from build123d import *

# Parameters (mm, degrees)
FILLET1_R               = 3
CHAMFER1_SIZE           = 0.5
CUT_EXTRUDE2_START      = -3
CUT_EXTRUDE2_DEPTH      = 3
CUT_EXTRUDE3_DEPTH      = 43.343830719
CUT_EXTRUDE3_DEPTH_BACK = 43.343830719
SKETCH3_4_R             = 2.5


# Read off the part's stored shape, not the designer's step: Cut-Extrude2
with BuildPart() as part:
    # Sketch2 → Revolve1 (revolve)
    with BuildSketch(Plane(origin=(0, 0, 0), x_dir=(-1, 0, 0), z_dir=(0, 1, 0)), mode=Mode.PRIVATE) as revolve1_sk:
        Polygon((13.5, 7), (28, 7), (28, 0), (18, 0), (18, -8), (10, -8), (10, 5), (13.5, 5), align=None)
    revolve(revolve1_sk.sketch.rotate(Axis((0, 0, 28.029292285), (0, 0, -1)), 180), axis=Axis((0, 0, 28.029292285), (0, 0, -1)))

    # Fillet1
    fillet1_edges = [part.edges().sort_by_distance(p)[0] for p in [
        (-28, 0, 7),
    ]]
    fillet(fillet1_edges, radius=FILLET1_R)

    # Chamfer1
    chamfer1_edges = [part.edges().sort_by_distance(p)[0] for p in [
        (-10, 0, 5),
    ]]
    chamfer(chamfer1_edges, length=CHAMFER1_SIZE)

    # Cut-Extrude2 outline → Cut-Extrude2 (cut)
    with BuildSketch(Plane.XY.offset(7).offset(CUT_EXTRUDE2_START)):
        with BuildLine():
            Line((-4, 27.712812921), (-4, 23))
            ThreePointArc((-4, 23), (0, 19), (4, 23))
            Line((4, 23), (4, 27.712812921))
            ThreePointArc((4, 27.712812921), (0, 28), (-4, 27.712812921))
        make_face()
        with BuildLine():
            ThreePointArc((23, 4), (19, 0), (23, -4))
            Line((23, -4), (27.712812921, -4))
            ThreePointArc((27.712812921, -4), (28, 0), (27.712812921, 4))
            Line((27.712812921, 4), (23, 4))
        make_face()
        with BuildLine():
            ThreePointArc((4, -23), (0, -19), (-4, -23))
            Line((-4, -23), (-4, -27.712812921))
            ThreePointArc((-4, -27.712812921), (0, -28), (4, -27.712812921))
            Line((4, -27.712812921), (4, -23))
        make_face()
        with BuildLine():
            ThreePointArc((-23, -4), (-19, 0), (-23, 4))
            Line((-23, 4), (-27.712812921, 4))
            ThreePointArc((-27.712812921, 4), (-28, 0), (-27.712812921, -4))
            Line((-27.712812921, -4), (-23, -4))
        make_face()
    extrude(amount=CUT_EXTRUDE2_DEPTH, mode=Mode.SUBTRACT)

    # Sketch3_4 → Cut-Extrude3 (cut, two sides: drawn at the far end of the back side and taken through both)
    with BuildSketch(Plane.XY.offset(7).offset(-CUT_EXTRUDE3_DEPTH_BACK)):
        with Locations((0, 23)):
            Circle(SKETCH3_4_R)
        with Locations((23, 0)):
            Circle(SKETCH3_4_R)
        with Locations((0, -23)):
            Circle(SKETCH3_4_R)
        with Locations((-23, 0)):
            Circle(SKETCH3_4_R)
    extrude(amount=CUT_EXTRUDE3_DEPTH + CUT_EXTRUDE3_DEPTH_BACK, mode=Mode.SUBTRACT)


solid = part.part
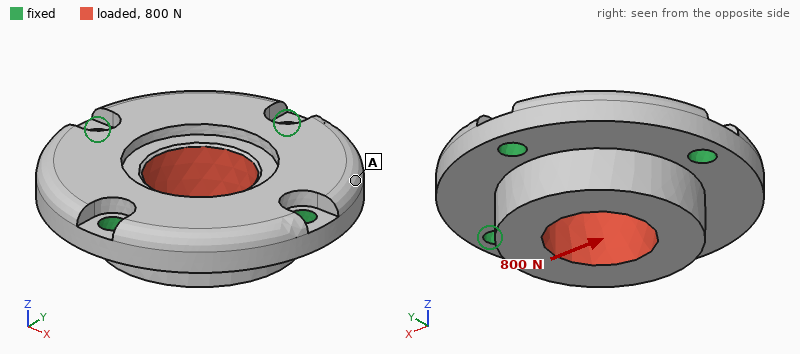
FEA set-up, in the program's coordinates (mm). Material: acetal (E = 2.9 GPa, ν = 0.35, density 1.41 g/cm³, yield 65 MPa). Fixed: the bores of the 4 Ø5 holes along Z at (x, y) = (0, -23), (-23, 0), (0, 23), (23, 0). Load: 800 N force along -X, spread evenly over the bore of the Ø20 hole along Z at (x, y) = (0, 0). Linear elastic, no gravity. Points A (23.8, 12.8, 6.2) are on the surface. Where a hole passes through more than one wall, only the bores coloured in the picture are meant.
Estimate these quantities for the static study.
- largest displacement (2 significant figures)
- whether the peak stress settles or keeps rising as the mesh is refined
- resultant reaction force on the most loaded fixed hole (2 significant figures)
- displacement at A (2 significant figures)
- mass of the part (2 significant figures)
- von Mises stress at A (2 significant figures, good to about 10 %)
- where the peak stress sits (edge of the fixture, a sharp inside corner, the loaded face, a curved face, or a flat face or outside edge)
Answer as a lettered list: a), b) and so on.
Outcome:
a) 24 µm
b) keeps rising
c) 230 N
d) 11 µm
e) 26 g
f) 1.3 MPa
g) edge of the fixture
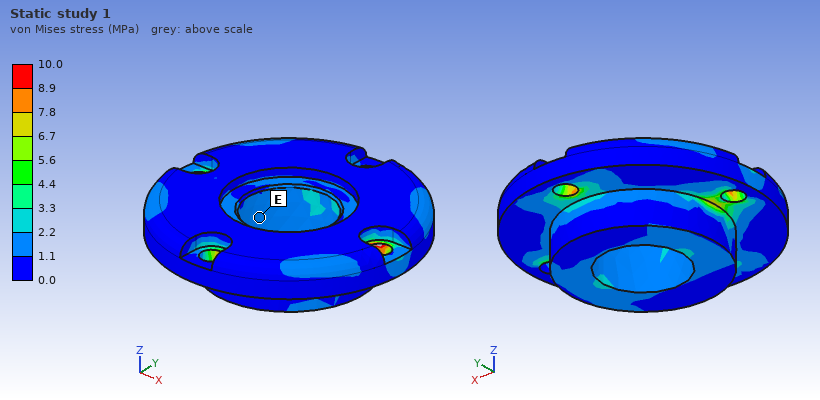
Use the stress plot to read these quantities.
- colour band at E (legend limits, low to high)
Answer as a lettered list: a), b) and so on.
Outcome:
a) 1.1 to 2.2 MPa
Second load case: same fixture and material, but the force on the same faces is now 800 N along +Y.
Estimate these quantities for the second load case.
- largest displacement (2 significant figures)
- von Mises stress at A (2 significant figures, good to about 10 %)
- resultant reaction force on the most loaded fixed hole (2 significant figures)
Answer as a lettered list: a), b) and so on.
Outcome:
a) 24 µm
b) 0.89 MPa
c) 230 N
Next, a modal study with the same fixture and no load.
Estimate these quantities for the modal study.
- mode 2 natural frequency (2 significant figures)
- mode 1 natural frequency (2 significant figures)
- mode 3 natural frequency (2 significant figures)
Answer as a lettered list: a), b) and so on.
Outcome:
a) 5800 Hz
b) 5500 Hz
c) 5900 Hz
